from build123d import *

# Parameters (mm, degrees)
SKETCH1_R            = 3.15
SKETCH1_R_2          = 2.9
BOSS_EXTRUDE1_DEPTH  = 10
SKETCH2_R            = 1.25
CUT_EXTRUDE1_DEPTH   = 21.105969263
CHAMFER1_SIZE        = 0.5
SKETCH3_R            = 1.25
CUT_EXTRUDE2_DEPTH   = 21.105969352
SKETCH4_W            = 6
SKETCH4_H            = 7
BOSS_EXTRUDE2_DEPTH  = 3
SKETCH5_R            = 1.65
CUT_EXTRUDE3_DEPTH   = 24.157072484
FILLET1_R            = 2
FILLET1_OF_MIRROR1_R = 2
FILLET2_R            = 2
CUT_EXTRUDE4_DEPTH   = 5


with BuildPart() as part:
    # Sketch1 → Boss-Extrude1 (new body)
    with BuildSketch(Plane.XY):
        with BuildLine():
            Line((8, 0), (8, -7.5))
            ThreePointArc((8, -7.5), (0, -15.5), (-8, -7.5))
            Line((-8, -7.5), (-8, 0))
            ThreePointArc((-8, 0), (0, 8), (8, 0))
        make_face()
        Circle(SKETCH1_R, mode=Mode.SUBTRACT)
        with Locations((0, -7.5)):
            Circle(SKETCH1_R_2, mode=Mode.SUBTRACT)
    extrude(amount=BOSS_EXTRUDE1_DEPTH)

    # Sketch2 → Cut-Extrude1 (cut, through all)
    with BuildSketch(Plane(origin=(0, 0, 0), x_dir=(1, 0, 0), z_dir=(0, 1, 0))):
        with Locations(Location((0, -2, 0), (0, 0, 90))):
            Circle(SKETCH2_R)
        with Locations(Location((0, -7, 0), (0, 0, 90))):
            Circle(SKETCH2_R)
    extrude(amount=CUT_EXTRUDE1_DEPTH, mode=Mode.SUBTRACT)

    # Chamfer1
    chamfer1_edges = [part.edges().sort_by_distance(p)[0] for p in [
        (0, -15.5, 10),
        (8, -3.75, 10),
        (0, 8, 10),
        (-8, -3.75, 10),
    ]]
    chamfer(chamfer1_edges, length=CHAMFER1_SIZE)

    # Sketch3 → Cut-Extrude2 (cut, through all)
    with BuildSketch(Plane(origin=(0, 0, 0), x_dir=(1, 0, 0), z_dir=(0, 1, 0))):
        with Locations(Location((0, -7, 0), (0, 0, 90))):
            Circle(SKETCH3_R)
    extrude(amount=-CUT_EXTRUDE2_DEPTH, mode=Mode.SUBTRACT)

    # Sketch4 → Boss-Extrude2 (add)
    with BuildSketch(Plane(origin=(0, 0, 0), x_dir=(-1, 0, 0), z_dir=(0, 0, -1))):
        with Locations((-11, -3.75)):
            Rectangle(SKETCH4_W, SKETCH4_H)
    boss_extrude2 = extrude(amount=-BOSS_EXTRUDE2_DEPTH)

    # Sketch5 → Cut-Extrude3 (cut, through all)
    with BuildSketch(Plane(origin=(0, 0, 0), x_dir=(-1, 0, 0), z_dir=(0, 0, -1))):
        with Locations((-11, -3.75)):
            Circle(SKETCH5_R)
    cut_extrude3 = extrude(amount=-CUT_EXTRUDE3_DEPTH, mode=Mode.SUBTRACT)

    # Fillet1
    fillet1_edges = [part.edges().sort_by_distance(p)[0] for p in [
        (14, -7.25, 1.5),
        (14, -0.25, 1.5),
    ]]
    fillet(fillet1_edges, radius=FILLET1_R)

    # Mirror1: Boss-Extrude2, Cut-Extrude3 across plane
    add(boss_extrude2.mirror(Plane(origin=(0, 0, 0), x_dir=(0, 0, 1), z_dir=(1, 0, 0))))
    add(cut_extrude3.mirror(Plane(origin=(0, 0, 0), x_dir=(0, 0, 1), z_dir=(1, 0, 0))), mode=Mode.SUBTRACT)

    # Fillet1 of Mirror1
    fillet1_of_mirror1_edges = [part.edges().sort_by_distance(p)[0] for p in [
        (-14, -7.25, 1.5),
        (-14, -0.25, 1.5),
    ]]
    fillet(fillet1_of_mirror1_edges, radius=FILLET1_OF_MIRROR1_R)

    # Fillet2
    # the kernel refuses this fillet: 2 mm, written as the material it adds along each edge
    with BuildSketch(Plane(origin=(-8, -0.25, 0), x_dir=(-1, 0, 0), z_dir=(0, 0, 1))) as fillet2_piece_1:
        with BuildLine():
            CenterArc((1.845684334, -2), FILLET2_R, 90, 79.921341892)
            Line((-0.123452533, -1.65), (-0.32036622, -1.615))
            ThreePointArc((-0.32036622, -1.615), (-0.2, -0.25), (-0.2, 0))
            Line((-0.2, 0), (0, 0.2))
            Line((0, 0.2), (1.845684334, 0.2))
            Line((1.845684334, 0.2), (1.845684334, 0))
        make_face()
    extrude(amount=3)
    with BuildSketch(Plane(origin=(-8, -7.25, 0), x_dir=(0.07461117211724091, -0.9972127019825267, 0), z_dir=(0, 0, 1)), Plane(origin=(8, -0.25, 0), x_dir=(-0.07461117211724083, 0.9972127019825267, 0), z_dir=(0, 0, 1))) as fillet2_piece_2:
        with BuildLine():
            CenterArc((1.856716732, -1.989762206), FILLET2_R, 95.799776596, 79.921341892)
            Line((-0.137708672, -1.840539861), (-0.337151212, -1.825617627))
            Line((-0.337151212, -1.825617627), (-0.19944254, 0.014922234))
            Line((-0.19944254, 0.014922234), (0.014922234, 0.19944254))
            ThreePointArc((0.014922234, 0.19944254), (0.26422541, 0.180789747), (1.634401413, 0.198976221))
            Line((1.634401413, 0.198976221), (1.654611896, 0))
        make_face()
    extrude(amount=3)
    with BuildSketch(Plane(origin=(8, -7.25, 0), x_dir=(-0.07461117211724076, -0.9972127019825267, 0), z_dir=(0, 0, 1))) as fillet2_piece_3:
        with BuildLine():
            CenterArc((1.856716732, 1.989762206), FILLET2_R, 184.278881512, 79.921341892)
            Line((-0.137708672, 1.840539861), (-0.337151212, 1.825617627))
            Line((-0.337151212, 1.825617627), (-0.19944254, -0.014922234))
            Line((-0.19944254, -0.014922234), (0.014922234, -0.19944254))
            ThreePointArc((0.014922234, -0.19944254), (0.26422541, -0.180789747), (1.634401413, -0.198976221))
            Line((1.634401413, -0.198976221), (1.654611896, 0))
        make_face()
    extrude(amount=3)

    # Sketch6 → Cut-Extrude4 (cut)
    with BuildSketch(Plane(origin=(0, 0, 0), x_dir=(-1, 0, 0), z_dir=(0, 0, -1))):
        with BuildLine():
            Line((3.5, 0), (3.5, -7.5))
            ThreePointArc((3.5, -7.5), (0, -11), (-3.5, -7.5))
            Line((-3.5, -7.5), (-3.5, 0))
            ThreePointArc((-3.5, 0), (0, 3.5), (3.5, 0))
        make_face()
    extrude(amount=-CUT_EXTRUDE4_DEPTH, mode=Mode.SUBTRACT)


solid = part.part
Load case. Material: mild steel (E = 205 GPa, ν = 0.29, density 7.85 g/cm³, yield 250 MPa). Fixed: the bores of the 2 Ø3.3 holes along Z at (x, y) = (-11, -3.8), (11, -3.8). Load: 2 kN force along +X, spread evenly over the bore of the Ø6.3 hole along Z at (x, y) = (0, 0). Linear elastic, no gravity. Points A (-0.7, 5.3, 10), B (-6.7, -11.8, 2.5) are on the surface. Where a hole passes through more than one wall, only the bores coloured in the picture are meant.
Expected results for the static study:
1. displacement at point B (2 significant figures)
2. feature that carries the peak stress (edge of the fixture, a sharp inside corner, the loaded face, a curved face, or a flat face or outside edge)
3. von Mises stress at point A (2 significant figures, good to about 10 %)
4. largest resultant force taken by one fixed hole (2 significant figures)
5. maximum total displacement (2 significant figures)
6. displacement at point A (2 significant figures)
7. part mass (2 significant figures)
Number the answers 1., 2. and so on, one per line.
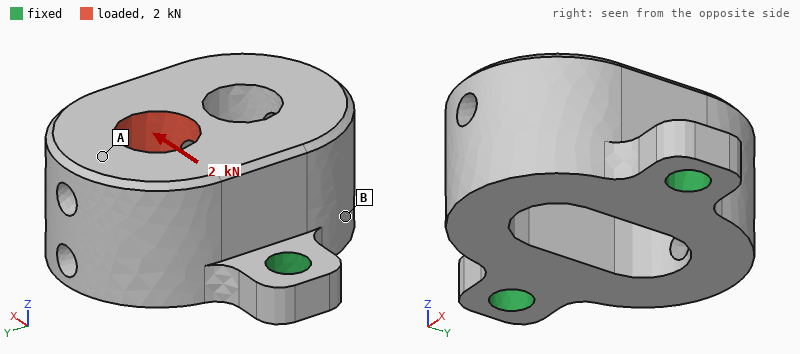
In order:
1. 1.4 µm
2. a curved face
3. 31 MPa
4. 1.2 kN
5. 6.5 µm
6. 5.6 µm
7. 20 g
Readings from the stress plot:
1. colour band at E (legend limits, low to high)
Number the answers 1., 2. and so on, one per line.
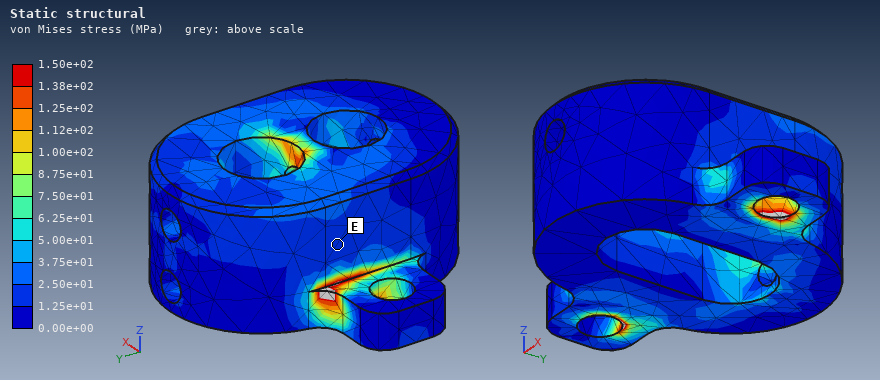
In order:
1. 1.25e+01 to 2.50e+01 MPa
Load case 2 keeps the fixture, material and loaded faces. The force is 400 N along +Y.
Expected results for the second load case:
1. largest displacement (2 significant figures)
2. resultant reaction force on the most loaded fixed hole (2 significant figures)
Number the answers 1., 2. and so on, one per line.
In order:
1. 10 µm
2. 200 N
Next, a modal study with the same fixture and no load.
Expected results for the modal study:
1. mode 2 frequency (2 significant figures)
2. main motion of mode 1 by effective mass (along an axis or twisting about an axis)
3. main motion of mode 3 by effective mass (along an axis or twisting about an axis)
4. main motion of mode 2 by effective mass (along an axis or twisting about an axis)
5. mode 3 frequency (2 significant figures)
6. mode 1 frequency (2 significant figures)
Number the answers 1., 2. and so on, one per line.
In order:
1. 25 kHz
2. along Y
3. along X
4. along Z
5. 33 kHz
6. 8700 Hz
